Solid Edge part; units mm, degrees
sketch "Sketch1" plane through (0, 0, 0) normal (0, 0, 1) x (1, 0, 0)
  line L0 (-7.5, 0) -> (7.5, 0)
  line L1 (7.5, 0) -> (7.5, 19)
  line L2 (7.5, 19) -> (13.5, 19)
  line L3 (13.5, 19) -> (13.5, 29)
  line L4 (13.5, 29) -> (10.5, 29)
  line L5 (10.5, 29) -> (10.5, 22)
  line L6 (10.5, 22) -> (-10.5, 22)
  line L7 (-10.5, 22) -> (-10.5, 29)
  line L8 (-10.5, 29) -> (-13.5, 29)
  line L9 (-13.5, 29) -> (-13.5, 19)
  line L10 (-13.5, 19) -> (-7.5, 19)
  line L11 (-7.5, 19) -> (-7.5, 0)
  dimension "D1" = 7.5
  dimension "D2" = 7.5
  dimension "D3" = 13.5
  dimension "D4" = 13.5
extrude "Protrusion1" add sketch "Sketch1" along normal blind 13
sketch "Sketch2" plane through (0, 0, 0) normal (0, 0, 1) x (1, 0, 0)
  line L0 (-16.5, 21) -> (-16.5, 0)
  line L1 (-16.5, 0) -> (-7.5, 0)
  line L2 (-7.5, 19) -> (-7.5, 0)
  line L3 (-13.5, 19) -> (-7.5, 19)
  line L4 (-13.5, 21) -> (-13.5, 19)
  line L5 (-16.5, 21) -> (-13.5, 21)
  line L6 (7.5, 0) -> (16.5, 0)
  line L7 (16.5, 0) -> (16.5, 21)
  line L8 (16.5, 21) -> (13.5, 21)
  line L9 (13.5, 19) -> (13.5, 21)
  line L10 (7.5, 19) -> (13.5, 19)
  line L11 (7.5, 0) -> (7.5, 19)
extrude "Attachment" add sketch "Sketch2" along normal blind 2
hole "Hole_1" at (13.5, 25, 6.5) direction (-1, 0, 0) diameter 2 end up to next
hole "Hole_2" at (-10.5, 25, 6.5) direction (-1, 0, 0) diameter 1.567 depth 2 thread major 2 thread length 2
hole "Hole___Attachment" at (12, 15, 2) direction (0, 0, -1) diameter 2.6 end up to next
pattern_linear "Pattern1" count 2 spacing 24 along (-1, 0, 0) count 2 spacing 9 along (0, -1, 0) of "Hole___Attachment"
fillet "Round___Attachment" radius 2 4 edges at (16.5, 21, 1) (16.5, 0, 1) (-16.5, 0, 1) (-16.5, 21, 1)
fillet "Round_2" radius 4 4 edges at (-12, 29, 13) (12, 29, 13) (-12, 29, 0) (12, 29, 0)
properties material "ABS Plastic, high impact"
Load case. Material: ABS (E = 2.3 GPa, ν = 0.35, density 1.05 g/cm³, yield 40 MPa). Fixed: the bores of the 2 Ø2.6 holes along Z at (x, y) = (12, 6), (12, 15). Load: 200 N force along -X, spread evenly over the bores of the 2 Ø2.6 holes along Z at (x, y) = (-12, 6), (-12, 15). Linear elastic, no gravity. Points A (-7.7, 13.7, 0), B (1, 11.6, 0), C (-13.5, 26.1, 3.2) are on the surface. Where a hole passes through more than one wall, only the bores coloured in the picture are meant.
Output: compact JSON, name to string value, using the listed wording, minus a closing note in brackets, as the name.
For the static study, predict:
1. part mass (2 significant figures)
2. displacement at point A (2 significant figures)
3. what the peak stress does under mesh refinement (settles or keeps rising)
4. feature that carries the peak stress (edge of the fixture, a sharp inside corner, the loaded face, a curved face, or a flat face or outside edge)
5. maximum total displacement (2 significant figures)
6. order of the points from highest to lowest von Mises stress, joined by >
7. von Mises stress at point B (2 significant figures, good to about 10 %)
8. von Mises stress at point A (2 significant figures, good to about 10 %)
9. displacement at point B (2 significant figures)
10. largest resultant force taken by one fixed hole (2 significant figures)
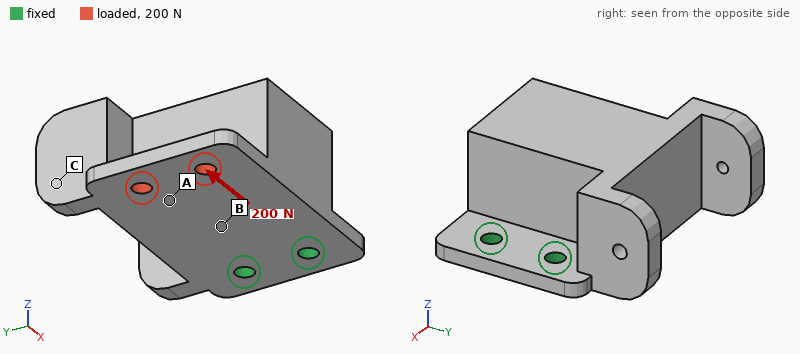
{"part mass": "6.2 g", "displacement at point A": "47 µm", "what the peak stress does under mesh refinement": "keeps rising", "feature that carries the peak stress": "edge of the fixture", "maximum total displacement": "83 µm", "order of the points from highest to lowest von Mises stress, joined by >": "A > B > C", "von Mises stress at point B": "3.5 MPa", "von Mises stress at point A": "5.4 MPa", "displacement at point B": "23 µm", "largest resultant force taken by one fixed hole": "100 N"}
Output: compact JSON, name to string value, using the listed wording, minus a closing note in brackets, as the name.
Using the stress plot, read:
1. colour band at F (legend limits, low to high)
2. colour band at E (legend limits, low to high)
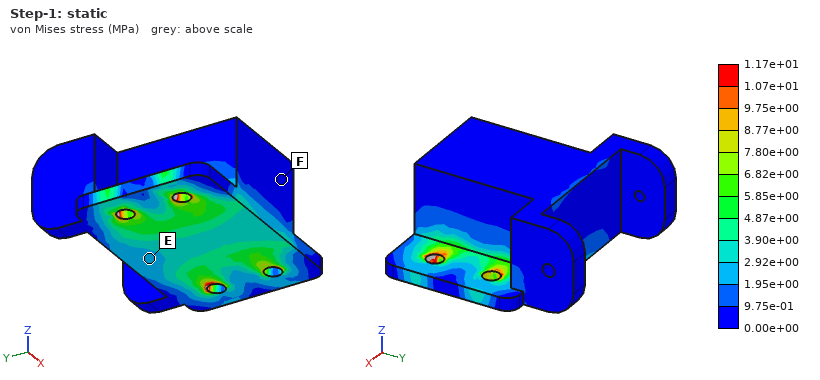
{"colour band at F": "0.00e+00 to 9.75e-01 MPa", "colour band at E": "1.95e+00 to 2.92e+00 MPa"}
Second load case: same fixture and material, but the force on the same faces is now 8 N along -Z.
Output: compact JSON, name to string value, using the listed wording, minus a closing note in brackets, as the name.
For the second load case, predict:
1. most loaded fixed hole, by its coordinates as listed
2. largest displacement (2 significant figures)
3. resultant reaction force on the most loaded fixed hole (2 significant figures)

{"most loaded fixed hole, by its coordinates as listed": "(12, 15)", "largest displacement": "0.45 mm", "resultant reaction force on the most loaded fixed hole": "5.4 N"}
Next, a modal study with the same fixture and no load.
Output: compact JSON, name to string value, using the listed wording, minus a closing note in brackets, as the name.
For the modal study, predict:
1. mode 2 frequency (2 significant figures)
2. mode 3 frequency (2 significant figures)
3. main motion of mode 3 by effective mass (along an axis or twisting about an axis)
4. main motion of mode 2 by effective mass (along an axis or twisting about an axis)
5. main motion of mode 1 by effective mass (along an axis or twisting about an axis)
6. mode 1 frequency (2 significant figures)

{"mode 2 frequency": "1700 Hz", "mode 3 frequency": "2300 Hz", "main motion of mode 3 by effective mass": "along Y", "main motion of mode 2 by effective mass": "along Y", "main motion of mode 1 by effective mass": "along Z", "mode 1 frequency": "480 Hz"}
